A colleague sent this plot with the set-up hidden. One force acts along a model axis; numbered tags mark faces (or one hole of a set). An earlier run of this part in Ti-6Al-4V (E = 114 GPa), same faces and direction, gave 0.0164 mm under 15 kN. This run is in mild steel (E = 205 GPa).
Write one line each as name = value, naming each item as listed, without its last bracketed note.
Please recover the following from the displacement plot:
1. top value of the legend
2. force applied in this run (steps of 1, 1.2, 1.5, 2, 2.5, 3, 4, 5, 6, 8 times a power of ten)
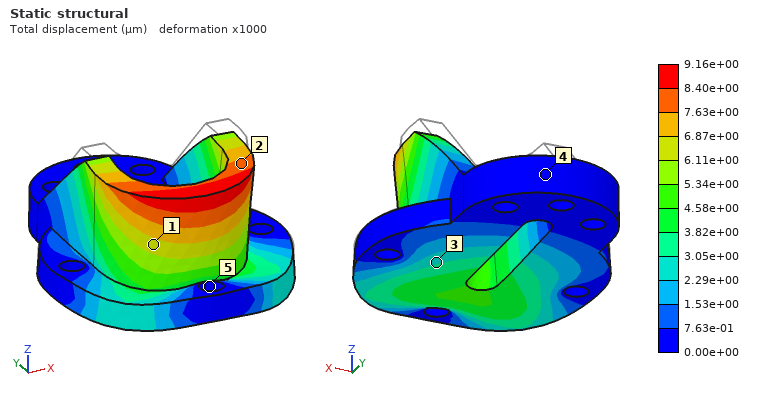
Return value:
top value of the legend = 9.16e+00 µm
force applied in this run = 15 kN
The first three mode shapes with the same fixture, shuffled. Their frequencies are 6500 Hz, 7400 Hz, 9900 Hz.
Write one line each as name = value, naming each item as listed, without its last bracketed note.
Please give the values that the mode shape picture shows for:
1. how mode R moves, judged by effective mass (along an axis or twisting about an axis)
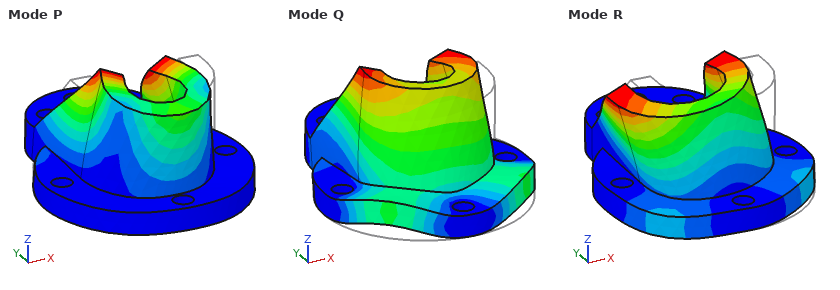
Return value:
how mode R moves, judged by effective mass = along X
